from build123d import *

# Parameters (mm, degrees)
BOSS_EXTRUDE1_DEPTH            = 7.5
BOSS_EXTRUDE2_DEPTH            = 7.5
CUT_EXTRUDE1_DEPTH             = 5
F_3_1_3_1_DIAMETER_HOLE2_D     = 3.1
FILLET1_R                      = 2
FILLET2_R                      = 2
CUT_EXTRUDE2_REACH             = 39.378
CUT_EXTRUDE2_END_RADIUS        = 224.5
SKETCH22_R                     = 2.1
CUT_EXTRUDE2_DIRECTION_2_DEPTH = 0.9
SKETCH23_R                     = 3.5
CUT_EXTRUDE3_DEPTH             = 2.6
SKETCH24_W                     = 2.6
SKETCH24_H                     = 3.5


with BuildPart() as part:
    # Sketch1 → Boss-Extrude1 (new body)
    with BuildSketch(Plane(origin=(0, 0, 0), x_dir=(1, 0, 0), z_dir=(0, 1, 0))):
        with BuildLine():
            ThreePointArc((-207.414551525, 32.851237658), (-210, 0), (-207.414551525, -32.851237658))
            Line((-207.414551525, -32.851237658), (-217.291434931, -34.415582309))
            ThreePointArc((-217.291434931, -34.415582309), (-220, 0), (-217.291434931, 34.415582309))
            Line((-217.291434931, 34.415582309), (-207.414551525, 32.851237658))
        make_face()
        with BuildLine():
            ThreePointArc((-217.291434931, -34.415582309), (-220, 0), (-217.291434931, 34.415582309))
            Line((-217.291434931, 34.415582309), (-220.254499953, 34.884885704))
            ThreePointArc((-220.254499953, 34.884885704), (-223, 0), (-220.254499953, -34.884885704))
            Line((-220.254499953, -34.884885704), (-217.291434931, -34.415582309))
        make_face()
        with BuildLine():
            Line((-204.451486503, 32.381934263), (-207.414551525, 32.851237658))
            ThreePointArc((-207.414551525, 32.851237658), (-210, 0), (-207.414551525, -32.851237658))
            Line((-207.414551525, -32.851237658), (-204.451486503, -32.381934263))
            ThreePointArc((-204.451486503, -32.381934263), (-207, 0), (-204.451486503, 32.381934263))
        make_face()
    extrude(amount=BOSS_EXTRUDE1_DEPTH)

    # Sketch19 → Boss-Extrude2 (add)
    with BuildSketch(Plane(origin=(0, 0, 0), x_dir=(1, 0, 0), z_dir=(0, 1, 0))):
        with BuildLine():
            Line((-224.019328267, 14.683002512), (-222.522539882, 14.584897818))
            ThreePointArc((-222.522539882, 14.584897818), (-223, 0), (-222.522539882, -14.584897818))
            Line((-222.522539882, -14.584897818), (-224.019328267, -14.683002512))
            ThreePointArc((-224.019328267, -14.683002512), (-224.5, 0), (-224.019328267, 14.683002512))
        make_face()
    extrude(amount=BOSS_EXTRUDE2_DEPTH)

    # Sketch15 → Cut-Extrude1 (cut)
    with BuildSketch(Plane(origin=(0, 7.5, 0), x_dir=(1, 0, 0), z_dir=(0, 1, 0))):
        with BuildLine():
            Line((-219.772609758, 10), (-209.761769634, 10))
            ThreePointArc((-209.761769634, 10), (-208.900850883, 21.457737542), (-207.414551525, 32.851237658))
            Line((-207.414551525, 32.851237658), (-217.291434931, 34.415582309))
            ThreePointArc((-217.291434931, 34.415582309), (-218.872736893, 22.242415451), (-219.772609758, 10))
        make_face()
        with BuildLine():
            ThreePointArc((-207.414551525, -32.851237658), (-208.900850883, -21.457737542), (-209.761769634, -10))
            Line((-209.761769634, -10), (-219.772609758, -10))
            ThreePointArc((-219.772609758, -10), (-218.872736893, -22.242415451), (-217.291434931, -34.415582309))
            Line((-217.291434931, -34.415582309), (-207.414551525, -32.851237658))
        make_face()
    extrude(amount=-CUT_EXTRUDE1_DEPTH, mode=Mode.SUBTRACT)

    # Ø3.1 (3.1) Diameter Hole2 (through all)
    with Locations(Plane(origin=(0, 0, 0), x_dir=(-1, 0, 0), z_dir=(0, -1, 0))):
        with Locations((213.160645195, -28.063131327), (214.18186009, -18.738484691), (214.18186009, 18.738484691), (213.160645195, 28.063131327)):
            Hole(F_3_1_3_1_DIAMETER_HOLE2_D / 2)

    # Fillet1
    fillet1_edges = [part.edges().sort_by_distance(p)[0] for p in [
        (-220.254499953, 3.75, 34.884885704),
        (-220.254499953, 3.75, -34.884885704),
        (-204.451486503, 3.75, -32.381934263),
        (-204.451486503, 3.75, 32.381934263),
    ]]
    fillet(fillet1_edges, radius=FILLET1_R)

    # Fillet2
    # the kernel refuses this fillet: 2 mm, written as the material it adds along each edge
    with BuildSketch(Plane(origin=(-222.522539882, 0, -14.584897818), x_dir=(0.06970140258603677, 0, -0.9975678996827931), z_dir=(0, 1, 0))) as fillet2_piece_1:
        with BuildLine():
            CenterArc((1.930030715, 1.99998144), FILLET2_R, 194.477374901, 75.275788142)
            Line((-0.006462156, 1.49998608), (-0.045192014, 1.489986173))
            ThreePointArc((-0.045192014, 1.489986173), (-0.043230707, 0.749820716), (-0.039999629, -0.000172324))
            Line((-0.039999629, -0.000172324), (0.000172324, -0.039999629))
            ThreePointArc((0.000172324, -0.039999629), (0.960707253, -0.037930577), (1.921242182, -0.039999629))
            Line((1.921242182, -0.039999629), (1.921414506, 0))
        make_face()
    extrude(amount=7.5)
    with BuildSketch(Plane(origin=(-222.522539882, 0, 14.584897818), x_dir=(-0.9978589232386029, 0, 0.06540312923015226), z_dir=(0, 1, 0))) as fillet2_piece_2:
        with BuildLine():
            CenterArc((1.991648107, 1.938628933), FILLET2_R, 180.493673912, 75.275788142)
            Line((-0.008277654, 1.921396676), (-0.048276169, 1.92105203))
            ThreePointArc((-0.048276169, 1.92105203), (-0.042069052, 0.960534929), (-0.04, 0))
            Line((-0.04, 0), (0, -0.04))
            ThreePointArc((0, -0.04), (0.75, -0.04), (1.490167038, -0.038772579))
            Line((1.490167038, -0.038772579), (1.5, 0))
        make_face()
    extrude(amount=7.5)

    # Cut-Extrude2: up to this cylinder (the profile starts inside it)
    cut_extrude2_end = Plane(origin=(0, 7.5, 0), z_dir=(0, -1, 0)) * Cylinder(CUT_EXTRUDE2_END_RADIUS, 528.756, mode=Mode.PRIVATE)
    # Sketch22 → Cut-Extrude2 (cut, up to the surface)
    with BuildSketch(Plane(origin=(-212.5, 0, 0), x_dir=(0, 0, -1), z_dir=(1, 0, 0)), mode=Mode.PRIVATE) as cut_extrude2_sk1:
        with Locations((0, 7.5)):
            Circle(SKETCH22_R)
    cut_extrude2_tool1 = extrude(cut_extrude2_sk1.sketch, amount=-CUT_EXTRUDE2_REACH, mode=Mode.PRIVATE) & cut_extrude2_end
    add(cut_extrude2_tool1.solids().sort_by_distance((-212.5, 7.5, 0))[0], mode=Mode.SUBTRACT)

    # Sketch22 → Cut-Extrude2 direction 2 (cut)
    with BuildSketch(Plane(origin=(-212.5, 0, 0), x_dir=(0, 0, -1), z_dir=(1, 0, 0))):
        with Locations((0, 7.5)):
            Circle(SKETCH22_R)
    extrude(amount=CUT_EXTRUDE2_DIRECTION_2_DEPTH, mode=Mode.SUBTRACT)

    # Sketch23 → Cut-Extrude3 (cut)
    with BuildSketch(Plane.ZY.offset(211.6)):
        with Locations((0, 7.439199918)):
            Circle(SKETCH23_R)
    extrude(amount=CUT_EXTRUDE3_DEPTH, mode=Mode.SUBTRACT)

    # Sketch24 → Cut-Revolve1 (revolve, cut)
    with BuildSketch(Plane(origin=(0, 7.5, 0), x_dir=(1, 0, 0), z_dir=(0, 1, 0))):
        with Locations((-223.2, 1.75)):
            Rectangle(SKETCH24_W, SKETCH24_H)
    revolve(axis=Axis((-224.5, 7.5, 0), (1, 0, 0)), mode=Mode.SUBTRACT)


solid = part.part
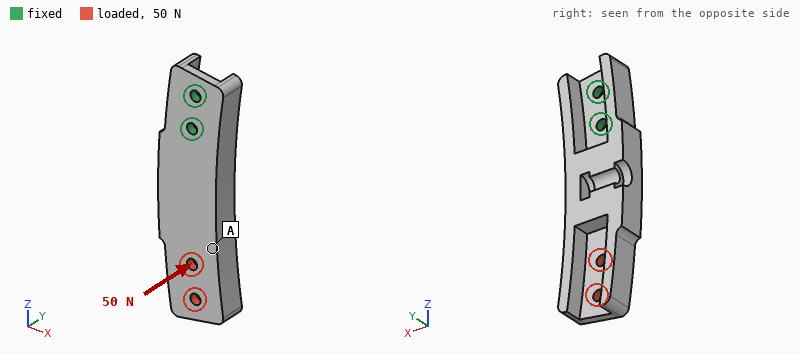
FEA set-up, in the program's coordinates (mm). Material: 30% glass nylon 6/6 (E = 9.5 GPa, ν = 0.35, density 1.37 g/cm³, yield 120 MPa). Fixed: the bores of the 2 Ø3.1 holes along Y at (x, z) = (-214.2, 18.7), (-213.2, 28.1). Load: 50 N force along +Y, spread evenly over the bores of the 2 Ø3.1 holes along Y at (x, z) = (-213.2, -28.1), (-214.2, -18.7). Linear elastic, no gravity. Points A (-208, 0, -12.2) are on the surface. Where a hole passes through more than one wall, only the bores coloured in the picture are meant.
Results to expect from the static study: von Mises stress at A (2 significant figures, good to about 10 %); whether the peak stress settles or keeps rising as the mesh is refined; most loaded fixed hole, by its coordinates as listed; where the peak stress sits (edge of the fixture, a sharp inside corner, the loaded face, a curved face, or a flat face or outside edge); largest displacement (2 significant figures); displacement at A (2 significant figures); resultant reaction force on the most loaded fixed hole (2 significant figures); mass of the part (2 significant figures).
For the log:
5.7 MPa
keeps rising
(-214.2, 18.7)
edge of the fixture
0.80 mm
0.41 mm
210 N
8.0 g
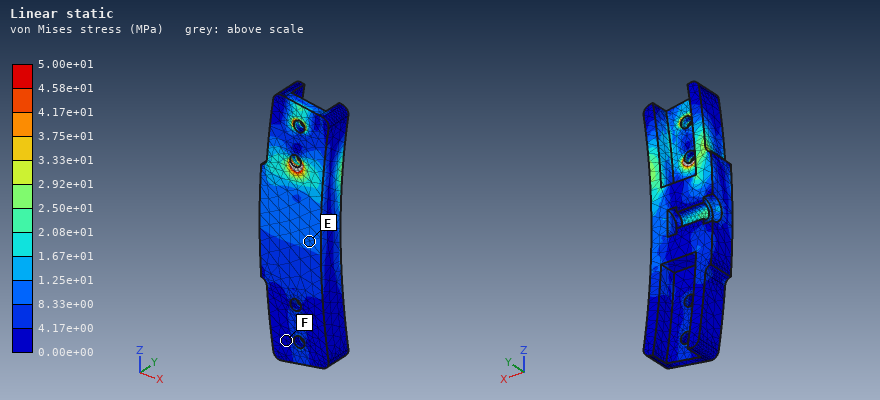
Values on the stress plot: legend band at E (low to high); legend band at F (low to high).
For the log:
8.33e+00 to 1.25e+01 MPa
0.00e+00 to 4.17e+00 MPa
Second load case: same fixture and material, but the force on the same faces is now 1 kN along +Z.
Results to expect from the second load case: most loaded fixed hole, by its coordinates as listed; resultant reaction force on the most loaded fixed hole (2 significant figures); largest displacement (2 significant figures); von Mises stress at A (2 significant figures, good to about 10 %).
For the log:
(-214.2, 18.7)
760 N
0.63 mm
31 MPa
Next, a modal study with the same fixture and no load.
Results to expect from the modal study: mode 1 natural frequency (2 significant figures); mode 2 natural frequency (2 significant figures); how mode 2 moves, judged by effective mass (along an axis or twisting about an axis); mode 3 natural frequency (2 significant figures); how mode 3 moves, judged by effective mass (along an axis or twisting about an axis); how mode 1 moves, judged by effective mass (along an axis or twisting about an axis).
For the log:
890 Hz
1800 Hz
along X
2800 Hz
twisting about Z
along Y
